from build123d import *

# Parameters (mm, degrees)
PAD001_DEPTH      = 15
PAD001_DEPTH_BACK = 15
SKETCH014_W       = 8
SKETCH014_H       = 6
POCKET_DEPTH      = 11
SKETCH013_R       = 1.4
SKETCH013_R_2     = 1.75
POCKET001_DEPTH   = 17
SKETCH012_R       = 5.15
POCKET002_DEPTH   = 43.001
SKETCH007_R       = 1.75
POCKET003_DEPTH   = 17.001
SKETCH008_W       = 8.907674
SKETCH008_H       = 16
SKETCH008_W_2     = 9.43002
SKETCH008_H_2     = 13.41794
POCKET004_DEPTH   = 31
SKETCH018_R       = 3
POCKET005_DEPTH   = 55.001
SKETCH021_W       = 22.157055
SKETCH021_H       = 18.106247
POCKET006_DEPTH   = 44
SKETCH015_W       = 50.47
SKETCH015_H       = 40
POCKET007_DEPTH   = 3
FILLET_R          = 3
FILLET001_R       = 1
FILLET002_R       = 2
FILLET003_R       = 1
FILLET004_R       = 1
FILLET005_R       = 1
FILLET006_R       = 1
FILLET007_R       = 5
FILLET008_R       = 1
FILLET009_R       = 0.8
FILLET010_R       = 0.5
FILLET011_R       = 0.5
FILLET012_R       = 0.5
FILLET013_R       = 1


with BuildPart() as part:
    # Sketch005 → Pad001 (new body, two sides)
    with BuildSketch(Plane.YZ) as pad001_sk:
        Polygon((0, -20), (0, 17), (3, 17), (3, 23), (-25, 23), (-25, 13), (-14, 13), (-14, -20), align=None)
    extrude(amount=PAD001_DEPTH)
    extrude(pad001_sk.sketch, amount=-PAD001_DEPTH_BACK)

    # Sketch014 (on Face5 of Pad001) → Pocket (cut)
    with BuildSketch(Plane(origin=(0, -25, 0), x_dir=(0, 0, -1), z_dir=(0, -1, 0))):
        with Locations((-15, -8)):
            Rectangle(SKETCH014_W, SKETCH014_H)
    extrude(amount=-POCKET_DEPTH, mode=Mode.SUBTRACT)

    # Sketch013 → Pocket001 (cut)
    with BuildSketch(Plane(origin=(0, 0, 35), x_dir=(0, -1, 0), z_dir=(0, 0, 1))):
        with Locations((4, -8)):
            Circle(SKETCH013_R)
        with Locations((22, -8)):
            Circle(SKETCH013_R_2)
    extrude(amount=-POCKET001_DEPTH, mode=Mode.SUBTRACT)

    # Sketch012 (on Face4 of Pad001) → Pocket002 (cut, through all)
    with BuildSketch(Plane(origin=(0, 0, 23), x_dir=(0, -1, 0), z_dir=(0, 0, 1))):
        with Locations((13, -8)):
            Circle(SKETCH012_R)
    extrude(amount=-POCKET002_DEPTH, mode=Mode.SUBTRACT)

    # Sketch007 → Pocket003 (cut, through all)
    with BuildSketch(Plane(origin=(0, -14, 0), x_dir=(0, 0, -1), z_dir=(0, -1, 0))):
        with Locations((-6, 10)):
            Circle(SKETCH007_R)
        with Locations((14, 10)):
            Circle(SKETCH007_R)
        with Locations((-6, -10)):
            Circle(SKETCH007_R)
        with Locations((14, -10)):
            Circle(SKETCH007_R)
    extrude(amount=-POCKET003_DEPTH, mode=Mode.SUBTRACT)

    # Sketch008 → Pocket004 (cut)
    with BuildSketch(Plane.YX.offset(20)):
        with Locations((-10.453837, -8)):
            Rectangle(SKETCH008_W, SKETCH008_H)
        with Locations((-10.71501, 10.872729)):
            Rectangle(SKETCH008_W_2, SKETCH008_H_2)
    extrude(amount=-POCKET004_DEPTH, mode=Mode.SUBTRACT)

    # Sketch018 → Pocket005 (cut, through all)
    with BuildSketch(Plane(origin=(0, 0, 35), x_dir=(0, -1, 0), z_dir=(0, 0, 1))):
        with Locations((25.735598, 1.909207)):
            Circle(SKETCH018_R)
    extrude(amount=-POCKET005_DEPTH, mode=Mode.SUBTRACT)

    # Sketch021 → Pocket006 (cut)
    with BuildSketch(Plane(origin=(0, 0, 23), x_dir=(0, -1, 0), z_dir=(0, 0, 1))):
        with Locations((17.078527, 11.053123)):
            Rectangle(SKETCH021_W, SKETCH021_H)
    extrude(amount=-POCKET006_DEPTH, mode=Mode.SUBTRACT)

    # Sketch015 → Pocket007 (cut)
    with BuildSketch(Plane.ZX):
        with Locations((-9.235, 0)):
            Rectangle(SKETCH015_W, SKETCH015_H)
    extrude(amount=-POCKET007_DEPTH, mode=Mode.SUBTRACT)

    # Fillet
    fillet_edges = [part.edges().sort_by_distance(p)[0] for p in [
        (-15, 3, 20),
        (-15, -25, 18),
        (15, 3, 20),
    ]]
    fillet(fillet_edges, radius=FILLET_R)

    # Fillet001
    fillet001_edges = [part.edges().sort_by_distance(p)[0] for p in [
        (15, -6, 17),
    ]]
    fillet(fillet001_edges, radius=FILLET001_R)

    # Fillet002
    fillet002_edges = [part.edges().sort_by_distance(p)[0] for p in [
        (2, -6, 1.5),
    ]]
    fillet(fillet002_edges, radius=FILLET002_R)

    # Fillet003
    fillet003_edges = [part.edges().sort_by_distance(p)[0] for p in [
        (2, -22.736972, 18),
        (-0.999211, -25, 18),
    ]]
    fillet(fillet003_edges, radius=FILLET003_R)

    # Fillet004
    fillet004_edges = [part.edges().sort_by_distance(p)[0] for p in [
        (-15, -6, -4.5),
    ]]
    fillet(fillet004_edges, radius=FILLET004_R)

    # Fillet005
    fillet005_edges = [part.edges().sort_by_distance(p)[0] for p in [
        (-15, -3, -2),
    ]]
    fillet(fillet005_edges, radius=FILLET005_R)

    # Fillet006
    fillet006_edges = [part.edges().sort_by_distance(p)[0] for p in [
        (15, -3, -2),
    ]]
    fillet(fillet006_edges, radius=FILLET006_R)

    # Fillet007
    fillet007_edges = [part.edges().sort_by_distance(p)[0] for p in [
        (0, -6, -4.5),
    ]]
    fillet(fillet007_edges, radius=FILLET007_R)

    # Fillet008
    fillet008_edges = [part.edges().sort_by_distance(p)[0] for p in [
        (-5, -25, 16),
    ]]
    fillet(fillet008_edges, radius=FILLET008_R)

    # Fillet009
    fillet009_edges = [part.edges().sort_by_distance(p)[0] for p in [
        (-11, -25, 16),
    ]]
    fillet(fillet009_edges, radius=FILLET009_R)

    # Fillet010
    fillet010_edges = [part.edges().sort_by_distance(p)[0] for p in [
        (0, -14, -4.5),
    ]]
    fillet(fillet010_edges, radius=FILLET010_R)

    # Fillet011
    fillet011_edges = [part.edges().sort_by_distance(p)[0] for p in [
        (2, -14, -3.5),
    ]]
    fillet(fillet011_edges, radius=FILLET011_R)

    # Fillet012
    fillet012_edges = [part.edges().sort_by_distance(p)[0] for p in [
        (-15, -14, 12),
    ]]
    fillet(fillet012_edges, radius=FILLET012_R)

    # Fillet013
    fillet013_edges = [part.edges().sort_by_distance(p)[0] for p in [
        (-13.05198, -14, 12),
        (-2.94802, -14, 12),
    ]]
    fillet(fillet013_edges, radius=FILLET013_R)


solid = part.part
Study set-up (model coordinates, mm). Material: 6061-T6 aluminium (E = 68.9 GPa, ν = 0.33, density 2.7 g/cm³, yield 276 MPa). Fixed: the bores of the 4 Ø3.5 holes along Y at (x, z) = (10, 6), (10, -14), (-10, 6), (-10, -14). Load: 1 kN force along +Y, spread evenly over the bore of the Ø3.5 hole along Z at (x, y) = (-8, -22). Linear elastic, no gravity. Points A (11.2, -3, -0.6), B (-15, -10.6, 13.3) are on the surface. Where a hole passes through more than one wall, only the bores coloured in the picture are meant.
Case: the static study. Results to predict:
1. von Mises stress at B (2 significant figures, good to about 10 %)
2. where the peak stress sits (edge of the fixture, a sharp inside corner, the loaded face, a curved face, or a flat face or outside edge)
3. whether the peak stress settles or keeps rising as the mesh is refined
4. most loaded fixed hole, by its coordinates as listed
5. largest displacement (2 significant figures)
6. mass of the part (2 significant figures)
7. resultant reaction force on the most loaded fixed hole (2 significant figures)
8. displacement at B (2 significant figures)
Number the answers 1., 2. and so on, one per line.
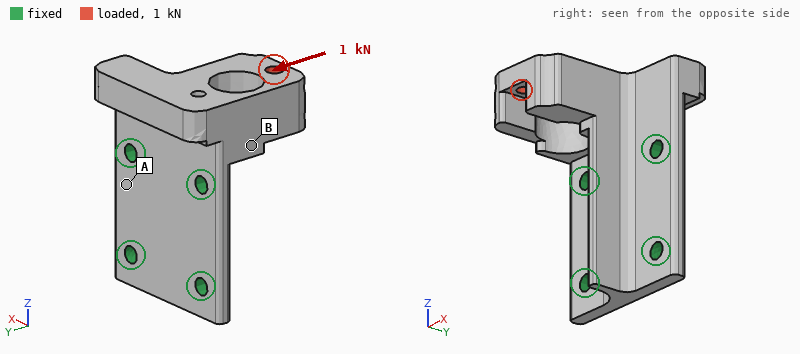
1. 38 MPa
2. edge of the fixture
3. keeps rising
4. (-10, 6)
5. 0.17 mm
6. 21 g
7. 1.2 kN
8. 0.059 mm
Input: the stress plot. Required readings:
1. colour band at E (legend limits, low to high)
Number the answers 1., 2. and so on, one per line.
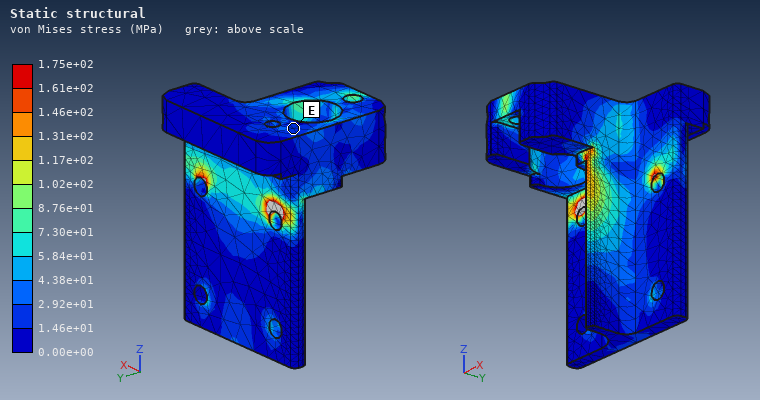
1. 1.46e+01 to 2.92e+01 MPa
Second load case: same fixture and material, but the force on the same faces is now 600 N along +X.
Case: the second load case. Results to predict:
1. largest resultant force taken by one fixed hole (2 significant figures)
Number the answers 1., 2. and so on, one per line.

1. 720 N
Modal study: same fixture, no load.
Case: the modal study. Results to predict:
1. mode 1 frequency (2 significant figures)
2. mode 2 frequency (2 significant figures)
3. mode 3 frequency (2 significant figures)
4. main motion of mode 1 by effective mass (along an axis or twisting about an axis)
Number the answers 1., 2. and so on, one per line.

1. 5100 Hz
2. 8100 Hz
3. 16 kHz
4. along Y
